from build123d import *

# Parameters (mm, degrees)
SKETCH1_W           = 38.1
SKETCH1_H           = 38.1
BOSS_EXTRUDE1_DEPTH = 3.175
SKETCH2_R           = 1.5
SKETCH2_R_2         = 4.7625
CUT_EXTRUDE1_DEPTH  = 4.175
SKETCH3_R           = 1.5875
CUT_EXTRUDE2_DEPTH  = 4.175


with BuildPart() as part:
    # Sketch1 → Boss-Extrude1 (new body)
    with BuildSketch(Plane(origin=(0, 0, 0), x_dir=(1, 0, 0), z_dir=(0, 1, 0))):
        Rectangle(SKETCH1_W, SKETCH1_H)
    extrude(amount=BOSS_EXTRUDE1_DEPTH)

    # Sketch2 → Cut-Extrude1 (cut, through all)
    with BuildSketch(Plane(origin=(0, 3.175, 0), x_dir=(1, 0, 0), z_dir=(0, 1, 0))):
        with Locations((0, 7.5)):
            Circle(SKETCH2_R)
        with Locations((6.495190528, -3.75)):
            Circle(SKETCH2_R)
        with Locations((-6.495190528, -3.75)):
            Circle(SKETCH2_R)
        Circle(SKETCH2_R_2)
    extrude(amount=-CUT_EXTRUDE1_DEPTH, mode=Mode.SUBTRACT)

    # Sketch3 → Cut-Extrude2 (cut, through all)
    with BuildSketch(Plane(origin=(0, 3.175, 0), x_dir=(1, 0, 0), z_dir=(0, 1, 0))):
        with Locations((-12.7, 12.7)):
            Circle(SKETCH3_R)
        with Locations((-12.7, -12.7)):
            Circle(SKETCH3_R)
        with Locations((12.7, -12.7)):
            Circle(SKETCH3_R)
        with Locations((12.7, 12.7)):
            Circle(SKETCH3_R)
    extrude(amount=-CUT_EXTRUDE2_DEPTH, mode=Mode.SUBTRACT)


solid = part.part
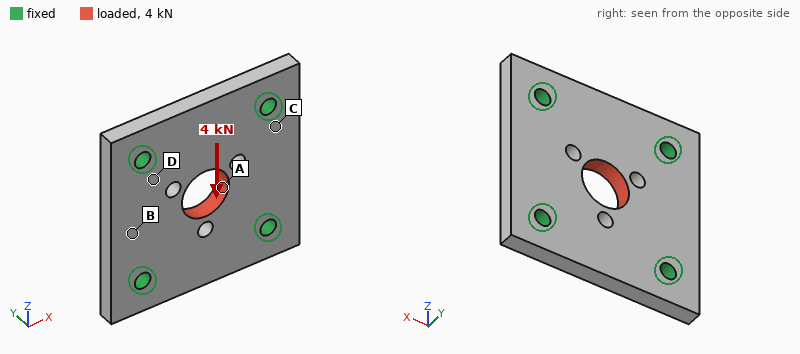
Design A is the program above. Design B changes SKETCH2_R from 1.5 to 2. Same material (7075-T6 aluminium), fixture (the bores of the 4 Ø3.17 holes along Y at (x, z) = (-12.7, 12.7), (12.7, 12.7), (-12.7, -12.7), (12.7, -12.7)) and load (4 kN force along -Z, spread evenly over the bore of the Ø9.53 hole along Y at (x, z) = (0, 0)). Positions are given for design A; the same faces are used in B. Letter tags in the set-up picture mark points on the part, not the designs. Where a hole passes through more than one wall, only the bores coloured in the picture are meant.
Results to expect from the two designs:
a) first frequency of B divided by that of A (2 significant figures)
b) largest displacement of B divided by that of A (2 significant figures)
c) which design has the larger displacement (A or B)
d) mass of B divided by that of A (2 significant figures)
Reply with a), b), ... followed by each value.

a) 1.0
b) 1.4
c) B
d) 0.99
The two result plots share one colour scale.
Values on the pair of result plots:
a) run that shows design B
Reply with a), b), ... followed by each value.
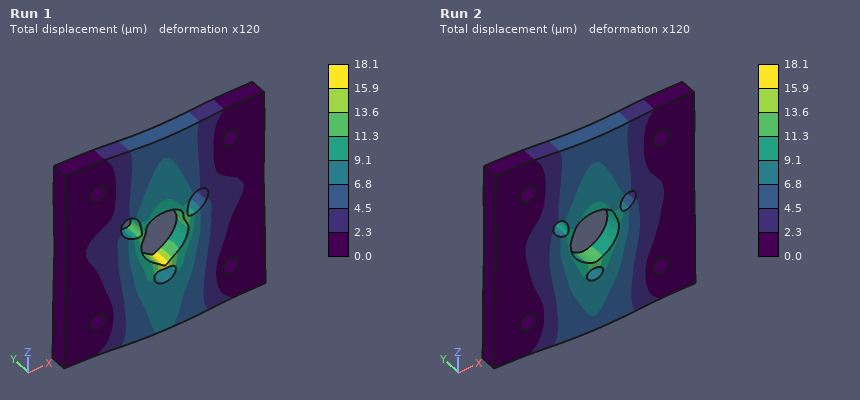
a) Run 1
